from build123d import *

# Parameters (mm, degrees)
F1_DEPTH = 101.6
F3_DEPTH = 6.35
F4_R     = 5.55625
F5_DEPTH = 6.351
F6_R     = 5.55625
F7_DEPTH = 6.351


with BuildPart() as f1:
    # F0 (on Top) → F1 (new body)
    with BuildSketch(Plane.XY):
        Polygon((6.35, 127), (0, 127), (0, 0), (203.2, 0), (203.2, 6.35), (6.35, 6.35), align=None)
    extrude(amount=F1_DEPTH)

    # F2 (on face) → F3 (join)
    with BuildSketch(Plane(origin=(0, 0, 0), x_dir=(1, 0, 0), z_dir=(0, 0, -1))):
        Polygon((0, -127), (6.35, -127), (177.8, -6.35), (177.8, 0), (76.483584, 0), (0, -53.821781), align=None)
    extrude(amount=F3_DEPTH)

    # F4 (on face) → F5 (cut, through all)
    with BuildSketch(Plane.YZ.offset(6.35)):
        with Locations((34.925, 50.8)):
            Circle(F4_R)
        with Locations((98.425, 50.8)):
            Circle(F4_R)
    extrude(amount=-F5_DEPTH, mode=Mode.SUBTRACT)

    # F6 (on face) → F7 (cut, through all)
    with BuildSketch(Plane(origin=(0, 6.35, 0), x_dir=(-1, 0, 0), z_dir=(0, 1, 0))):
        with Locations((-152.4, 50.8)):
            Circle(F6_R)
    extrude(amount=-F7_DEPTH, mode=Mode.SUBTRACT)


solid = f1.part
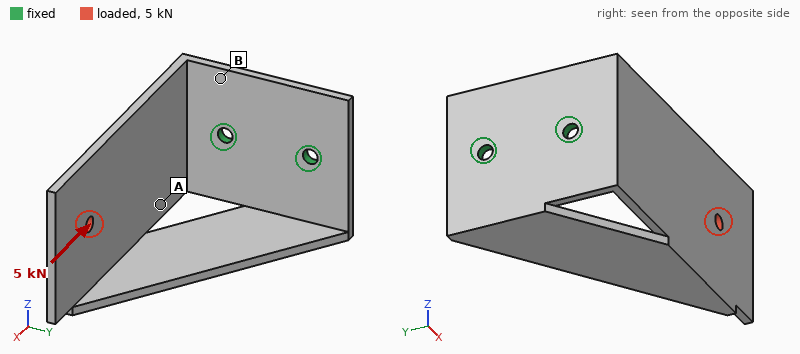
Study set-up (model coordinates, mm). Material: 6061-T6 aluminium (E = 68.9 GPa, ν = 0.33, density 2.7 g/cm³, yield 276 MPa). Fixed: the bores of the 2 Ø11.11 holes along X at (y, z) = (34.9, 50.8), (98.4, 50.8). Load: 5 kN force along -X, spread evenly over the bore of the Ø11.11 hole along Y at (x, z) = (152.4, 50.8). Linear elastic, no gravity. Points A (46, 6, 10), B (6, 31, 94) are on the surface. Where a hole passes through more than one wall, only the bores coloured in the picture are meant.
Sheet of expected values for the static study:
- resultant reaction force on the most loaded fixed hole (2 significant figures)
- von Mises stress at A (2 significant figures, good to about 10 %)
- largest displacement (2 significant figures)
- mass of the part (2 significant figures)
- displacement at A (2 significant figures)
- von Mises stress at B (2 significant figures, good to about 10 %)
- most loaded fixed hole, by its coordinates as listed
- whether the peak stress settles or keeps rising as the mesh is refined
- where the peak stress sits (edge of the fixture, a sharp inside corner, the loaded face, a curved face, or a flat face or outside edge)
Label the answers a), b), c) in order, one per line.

a) 6.0 kN
b) 24 MPa
c) 1.5 mm
d) 730 g
e) 0.44 mm
f) 57 MPa
g) (34.9, 50.8)
h) keeps rising
i) edge of the fixture
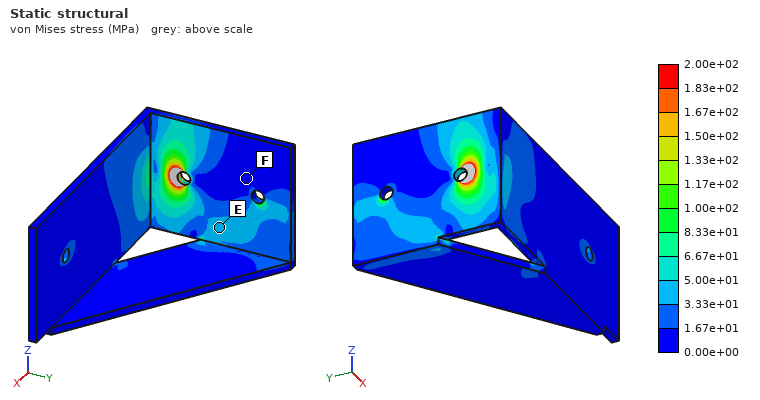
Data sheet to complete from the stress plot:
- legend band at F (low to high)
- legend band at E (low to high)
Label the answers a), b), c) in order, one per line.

a) 0.00e+00 to 1.67e+01 MPa
b) 3.33e+01 to 5.00e+01 MPa
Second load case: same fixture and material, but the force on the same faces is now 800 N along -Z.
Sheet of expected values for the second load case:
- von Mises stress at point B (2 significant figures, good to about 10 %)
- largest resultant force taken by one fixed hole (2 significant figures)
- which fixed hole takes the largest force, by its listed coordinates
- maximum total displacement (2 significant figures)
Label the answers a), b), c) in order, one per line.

a) 44 MPa
b) 1.1 kN
c) (34.9, 50.8)
d) 2.6 mm
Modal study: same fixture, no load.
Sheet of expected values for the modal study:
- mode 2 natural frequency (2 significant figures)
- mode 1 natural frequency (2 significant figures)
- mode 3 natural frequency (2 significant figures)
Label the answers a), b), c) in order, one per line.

a) 240 Hz
b) 190 Hz
c) 670 Hz
